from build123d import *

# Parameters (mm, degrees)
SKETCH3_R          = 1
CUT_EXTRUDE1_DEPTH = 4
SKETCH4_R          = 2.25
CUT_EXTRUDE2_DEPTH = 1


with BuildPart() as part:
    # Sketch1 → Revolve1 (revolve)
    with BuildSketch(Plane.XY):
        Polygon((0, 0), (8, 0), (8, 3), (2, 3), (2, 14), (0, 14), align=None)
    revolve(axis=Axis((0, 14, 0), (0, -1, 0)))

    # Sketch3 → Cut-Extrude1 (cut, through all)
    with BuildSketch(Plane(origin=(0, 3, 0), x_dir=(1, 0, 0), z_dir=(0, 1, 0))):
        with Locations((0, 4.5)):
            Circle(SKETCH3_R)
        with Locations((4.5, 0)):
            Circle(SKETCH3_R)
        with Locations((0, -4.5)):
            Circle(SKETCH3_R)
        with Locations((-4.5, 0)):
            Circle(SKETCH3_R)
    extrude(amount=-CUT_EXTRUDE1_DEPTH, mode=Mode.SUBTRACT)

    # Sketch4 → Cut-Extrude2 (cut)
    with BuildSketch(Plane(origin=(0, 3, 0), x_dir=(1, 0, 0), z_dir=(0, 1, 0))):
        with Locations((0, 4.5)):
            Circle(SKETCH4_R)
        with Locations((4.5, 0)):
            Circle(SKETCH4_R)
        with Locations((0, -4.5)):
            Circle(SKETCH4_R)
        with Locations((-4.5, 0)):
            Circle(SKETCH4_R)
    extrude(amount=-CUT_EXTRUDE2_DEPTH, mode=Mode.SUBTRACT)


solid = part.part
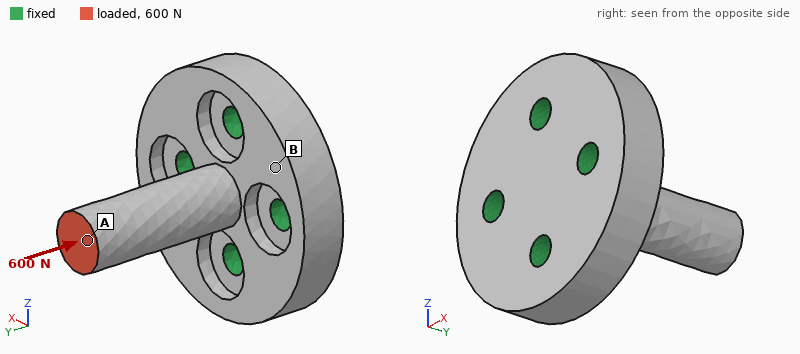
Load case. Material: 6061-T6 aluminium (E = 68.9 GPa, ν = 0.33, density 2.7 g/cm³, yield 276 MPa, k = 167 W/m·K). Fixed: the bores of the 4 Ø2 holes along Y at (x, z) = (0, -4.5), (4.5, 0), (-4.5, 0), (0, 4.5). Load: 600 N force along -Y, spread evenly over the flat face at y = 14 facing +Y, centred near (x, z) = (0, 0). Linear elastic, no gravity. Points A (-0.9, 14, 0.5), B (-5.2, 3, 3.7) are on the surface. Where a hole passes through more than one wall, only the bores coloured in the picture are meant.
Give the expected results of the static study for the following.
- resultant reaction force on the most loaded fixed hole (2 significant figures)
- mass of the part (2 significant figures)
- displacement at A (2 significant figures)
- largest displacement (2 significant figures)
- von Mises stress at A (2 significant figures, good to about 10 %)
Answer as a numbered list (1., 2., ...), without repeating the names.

1. 160 N
2. 1.8 g
3. 10 µm
4. 10 µm
5. 48 MPa
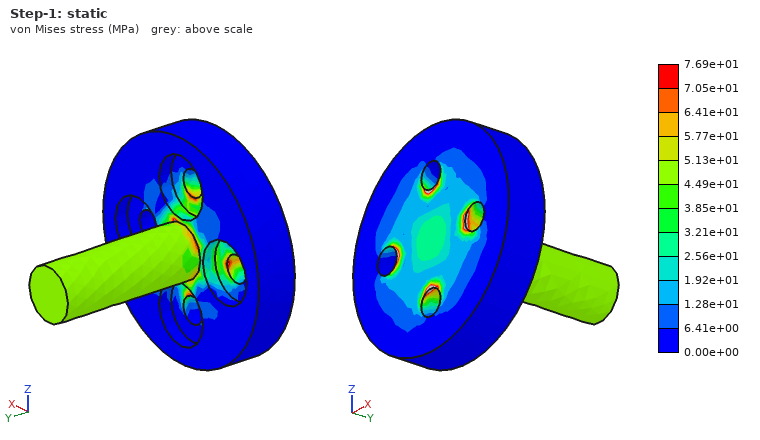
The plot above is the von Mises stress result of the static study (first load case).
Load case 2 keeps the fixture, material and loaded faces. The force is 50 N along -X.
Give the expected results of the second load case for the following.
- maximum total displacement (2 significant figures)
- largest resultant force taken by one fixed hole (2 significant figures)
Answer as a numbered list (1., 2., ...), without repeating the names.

1. 37 µm
2. 79 N
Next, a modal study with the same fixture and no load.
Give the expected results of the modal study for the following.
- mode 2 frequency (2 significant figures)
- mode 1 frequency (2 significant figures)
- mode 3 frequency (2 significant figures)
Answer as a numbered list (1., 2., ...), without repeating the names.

1. 18 kHz
2. 18 kHz
3. 66 kHz
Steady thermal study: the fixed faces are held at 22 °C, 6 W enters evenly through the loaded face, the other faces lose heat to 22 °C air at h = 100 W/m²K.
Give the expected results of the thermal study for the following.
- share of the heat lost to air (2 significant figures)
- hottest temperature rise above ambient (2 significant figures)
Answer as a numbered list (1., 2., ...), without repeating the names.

1. 5.0 %
2. 35 K
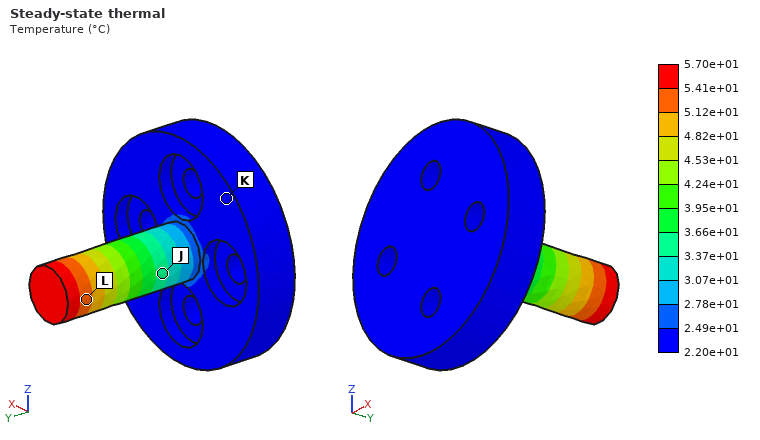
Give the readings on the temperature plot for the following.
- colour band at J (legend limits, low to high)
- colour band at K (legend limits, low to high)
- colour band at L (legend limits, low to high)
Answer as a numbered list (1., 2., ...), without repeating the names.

1. 3.37e+01 to 3.66e+01 °C
2. 2.20e+01 to 2.49e+01 °C
3. 5.12e+01 to 5.41e+01 °C
